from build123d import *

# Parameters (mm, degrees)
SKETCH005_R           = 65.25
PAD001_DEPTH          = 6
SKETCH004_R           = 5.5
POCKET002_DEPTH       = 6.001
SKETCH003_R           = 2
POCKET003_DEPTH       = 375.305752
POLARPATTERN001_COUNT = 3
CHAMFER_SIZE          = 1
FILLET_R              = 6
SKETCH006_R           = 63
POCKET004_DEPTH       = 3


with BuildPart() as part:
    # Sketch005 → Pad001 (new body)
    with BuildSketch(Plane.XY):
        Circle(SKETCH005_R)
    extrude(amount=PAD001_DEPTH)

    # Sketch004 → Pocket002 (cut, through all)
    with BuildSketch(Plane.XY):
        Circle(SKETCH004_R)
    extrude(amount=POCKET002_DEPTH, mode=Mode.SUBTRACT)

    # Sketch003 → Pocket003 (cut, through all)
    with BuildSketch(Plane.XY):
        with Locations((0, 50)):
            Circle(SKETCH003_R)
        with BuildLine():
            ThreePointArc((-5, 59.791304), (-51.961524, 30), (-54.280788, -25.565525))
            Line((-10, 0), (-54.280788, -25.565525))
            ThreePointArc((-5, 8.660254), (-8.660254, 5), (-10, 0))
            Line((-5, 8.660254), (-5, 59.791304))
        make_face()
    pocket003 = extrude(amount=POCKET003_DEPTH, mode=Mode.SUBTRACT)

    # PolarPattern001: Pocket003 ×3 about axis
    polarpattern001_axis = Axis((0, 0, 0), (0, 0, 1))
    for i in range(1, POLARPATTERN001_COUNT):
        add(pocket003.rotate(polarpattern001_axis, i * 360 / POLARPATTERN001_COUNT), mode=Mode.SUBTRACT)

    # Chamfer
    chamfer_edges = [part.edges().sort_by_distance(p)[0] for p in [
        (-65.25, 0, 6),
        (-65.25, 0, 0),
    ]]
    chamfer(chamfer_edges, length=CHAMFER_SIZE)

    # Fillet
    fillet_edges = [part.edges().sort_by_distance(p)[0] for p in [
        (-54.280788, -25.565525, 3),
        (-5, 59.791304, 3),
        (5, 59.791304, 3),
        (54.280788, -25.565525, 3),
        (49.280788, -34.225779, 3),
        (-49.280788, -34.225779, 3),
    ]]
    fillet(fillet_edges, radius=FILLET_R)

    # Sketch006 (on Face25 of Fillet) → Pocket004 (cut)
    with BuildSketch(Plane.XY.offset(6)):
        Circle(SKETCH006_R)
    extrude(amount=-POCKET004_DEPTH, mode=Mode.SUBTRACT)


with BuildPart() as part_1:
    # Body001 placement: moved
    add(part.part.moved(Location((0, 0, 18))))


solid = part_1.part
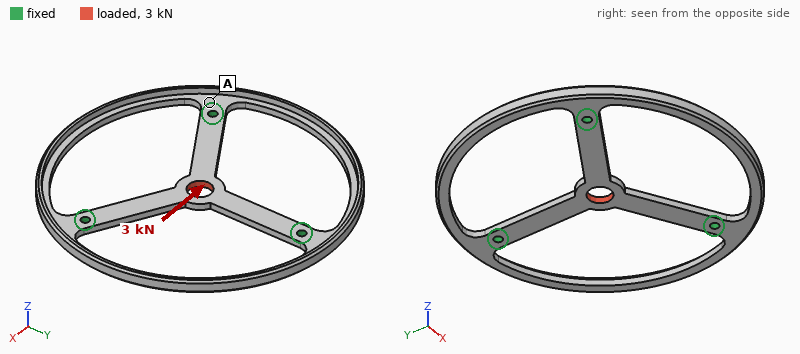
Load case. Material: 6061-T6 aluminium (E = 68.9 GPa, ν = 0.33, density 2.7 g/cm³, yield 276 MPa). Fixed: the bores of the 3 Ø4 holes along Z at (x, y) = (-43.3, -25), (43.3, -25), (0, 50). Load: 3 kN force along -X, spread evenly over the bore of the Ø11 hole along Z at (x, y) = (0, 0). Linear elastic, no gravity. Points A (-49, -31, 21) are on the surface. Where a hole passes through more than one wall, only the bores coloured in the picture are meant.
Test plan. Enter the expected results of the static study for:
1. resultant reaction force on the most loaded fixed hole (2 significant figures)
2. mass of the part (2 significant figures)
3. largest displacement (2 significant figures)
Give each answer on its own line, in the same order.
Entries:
1.7 kN
37 g
79 µm
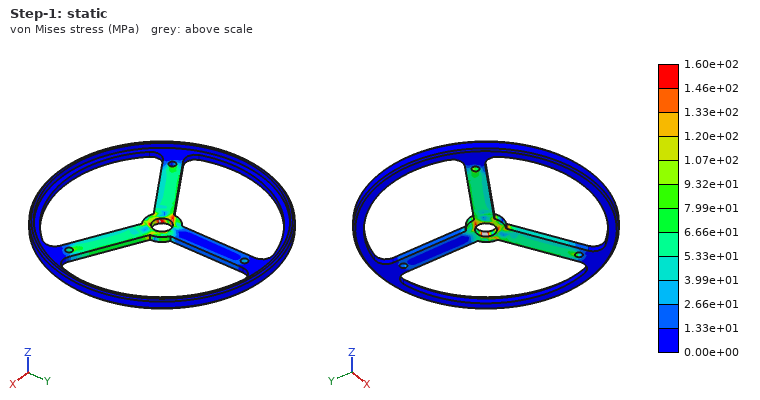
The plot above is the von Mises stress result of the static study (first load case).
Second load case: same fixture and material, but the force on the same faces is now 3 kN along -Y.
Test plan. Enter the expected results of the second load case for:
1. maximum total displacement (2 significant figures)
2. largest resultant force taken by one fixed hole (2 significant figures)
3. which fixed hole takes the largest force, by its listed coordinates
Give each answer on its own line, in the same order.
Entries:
82 µm
2.0 kN
(0, 50)
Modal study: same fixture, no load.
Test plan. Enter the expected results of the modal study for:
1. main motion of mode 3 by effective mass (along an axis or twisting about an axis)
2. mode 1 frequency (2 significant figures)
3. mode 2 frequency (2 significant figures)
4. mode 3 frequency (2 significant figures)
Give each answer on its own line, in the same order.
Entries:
along Z
970 Hz
970 Hz
1400 Hz
